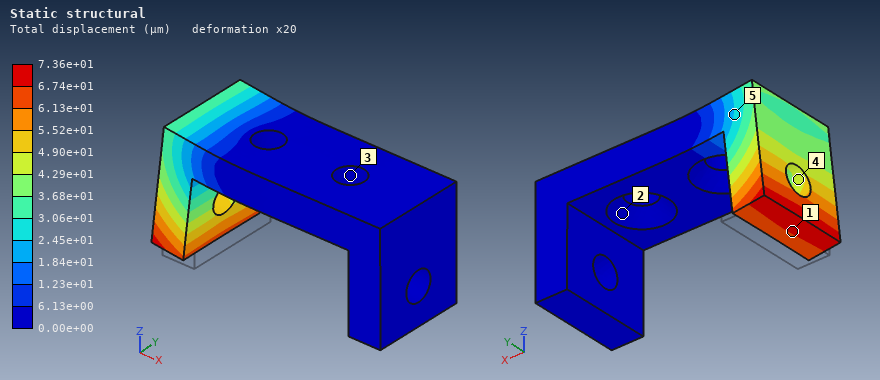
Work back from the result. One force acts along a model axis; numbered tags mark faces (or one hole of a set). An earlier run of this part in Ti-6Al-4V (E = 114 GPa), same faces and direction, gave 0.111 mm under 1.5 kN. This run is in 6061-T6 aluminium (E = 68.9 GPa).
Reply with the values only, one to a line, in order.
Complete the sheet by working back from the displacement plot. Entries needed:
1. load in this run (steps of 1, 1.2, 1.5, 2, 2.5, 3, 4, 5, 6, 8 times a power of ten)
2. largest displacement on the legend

600 N
7.36e+01 µm
